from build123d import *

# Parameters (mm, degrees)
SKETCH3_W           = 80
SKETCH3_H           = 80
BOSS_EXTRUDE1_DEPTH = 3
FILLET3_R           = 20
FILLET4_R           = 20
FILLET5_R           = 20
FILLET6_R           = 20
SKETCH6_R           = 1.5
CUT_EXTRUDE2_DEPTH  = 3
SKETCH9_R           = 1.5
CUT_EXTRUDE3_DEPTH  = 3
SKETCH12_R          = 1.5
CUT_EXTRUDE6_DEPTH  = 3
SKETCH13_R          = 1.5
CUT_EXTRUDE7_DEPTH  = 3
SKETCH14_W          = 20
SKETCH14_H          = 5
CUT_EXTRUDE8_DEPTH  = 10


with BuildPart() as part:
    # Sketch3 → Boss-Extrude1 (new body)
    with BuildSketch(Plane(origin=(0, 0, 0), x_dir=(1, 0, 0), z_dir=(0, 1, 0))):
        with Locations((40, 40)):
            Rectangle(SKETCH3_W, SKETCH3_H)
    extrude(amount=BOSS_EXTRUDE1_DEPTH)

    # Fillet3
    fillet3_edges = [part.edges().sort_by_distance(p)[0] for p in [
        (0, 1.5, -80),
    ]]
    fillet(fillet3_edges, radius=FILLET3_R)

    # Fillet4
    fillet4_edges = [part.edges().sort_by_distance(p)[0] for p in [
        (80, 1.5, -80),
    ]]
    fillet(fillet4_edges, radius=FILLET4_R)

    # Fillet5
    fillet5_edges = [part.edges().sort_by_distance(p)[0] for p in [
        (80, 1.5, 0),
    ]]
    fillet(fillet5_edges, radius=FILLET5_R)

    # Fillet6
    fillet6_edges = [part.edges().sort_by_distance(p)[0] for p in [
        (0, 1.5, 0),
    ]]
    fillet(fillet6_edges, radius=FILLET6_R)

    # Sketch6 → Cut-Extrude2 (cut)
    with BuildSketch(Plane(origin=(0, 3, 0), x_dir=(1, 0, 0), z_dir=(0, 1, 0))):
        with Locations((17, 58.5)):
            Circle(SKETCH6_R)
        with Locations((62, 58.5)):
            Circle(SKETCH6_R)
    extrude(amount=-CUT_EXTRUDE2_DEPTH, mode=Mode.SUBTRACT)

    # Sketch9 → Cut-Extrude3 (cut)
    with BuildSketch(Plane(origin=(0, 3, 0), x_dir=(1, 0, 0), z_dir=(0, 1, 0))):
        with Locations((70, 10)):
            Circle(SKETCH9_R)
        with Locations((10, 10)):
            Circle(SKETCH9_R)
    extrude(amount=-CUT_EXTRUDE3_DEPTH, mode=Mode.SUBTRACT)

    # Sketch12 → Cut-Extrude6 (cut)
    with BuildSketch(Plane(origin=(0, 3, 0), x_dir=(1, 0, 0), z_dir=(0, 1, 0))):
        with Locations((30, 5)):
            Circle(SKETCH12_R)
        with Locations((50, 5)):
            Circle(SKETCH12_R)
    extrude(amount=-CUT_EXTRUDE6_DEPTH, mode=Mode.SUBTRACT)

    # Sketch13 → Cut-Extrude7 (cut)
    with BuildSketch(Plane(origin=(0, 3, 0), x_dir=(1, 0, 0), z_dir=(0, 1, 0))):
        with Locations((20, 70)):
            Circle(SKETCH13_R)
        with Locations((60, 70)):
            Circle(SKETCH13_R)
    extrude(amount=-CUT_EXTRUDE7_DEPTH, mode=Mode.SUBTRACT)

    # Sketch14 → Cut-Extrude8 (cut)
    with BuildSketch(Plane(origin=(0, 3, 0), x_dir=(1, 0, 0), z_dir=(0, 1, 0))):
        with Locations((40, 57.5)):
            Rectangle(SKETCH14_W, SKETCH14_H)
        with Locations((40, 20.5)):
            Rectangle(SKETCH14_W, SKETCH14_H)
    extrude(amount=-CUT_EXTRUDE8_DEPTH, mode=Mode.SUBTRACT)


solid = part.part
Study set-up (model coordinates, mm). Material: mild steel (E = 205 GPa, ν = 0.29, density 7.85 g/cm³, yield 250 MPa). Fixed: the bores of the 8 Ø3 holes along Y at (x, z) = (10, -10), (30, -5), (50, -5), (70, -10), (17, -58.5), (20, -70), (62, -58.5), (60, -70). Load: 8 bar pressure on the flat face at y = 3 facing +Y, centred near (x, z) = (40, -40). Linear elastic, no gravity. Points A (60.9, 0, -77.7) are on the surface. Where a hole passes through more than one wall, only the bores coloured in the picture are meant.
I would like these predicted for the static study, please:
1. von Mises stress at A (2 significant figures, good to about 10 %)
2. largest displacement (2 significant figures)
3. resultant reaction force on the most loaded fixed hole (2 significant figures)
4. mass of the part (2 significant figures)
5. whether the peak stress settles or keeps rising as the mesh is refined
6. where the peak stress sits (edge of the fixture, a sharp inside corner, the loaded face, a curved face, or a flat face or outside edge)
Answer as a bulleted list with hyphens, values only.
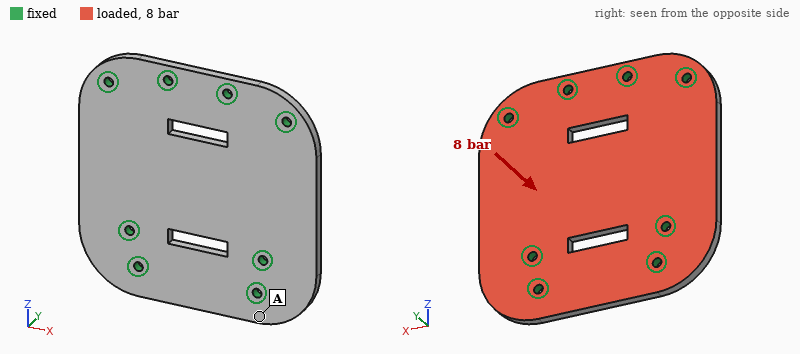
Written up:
- 31 MPa
- 49 µm
- 1.1 kN
- 140 g
- keeps rising
- edge of the fixture
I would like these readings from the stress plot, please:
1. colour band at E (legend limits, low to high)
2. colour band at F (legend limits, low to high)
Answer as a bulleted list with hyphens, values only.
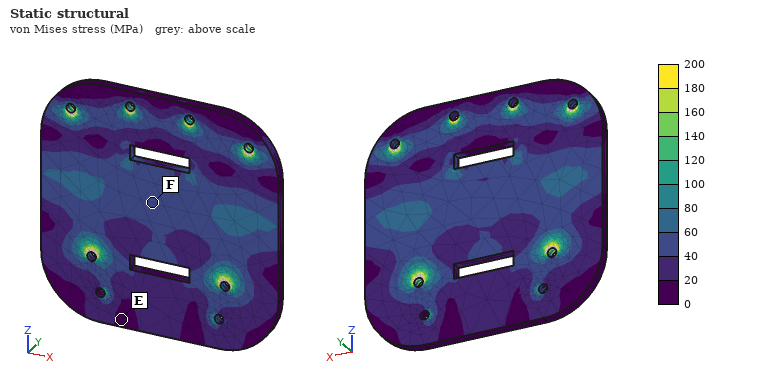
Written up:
- 0 to 20 MPa
- 40 to 60 MPa
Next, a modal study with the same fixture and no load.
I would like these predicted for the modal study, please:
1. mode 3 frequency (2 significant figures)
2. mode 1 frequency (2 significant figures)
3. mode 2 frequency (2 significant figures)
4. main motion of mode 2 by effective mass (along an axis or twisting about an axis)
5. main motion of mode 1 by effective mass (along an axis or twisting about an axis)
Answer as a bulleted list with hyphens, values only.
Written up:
- 6000 Hz
- 5000 Hz
- 5700 Hz
- twisting about Z
- along Y
